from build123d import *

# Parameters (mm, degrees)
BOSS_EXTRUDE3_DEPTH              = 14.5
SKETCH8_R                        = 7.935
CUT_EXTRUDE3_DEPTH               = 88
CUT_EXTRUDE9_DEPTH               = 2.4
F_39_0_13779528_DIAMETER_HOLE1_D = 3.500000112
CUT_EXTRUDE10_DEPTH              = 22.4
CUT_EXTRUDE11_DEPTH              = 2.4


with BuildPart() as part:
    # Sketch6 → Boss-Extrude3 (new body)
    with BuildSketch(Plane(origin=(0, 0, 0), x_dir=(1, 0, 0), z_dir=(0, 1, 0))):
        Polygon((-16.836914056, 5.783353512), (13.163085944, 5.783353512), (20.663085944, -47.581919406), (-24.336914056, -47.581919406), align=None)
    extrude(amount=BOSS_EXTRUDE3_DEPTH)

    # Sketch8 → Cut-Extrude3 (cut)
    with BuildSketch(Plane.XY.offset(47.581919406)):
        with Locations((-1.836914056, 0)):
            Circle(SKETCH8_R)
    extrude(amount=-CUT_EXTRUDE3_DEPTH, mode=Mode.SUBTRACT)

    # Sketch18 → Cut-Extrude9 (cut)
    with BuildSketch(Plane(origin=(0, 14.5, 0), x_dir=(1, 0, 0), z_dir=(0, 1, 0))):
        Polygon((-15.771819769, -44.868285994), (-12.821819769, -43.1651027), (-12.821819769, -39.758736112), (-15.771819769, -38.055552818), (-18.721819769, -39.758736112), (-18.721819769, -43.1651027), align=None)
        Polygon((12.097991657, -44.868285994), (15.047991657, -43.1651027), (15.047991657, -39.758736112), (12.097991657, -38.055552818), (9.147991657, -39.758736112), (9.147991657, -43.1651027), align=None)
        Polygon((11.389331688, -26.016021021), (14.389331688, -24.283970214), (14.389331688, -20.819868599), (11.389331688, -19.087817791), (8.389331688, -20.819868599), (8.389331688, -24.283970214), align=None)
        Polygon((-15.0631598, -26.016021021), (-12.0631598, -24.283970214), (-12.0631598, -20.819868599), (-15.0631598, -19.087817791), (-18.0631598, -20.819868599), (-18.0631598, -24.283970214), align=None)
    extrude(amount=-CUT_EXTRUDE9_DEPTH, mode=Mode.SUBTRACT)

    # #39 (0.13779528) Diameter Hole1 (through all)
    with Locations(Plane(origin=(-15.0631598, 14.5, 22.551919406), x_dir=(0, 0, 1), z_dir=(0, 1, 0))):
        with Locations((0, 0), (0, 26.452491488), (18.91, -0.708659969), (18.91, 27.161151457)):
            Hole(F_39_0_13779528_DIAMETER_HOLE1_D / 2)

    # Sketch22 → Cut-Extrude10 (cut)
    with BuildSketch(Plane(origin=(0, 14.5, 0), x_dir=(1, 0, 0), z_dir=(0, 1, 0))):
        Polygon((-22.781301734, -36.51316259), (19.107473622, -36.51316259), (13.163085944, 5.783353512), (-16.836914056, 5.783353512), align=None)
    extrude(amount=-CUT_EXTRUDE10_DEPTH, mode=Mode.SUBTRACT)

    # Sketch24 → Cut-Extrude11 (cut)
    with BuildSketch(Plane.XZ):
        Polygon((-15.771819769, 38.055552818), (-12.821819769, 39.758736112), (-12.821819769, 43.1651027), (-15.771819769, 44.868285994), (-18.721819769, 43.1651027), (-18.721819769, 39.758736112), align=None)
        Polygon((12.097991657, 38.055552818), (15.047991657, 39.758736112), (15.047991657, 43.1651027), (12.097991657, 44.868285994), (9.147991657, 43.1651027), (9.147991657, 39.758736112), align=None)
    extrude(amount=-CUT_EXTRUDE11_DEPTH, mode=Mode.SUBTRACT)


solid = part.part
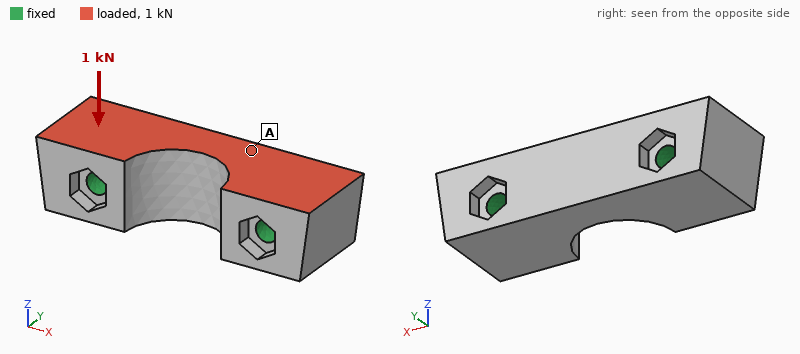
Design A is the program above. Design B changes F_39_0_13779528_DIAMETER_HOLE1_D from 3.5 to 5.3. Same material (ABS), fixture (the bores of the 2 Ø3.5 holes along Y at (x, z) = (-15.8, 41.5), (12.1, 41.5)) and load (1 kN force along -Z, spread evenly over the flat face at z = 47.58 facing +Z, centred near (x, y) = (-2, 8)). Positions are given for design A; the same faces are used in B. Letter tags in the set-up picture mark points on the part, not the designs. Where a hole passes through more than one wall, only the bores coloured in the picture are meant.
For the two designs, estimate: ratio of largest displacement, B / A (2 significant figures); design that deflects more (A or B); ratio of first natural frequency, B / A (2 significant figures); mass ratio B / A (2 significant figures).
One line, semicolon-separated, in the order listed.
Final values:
0.80; A; 1.3; 0.96
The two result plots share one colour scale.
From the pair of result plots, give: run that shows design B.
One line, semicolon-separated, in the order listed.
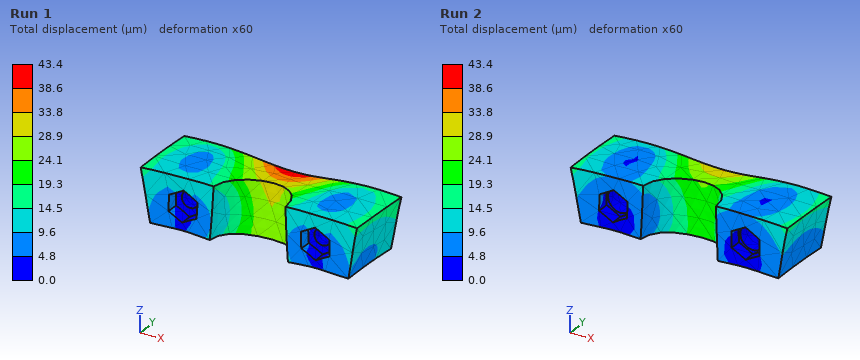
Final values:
Run 2
